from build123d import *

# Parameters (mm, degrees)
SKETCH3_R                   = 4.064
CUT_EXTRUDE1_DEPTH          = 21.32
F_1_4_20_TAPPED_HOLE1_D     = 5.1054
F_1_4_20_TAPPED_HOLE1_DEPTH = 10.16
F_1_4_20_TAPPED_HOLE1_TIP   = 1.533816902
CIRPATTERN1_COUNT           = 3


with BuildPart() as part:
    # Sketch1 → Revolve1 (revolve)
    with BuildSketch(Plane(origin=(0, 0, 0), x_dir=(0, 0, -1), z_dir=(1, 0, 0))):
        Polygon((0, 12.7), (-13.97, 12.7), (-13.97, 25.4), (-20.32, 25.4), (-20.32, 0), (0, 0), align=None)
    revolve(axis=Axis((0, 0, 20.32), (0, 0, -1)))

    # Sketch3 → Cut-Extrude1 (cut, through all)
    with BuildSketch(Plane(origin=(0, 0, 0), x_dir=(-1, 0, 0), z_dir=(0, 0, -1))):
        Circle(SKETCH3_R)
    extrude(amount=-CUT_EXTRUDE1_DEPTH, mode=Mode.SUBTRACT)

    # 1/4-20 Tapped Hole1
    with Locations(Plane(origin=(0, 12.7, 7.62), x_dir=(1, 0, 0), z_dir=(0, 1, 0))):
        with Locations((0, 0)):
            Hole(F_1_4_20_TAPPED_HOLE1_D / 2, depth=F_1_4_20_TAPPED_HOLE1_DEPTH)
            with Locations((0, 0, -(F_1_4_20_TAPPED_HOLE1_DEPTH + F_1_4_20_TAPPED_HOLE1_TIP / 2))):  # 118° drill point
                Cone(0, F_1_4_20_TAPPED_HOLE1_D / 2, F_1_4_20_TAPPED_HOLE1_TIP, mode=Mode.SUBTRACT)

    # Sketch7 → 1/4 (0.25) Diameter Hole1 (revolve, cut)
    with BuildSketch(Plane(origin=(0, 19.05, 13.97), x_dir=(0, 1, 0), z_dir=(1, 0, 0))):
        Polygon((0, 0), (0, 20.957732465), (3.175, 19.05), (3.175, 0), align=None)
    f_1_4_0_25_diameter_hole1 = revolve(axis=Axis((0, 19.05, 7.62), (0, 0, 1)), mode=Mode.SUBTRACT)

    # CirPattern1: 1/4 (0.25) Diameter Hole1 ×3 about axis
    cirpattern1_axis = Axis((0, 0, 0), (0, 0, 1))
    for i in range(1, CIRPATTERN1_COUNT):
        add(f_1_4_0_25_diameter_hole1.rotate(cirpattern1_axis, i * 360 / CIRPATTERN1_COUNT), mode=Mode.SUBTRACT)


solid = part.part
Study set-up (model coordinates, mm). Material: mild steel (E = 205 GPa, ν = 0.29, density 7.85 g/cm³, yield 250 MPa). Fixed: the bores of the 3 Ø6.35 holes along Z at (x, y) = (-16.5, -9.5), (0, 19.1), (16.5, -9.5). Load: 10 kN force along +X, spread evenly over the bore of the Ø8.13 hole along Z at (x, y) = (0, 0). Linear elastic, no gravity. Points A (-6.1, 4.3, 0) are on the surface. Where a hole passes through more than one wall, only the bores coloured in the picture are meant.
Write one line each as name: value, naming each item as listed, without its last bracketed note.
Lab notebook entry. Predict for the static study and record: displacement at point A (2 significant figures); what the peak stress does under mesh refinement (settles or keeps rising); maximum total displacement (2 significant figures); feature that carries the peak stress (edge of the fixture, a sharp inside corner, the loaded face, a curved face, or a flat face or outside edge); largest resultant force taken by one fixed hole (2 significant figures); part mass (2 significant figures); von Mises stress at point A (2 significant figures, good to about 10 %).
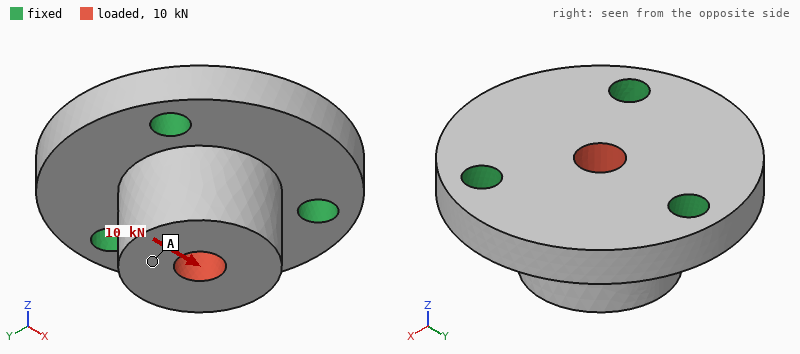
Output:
displacement at point A: 9.0 µm
what the peak stress does under mesh refinement: keeps rising
maximum total displacement: 9.6 µm
feature that carries the peak stress: edge of the fixture
largest resultant force taken by one fixed hole: 4.3 kN
part mass: 140 g
von Mises stress at point A: 17 MPa
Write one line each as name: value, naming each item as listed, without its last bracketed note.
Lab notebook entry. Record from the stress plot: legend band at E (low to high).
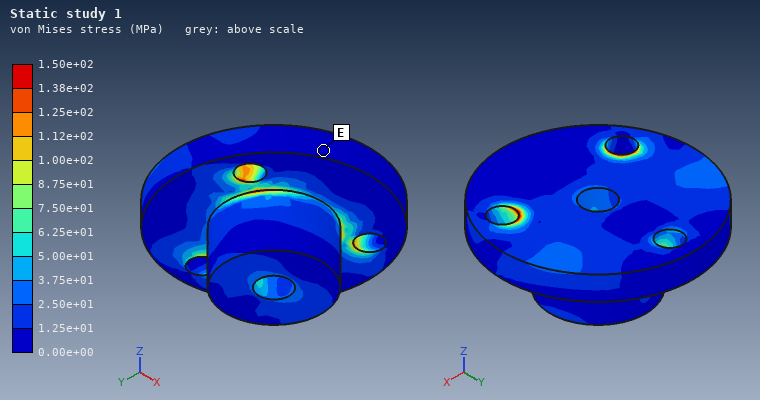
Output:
legend band at E: 0.00e+00 to 1.25e+01 MPa
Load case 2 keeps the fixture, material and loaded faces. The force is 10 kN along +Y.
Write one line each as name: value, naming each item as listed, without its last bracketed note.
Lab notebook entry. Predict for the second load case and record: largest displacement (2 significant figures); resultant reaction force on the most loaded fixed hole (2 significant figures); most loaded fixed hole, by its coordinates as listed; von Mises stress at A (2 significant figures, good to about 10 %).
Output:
largest displacement: 9.9 µm
resultant reaction force on the most loaded fixed hole: 4.7 kN
most loaded fixed hole, by its coordinates as listed: (0, 19.1)
von Mises stress at A: 16 MPa
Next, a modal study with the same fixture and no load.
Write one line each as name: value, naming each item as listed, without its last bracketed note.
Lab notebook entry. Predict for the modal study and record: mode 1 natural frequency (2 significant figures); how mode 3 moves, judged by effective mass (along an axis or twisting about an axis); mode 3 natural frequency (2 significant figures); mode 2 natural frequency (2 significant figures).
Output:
mode 1 natural frequency: 18 kHz
how mode 3 moves, judged by effective mass: along Z
mode 3 natural frequency: 21 kHz
mode 2 natural frequency: 18 kHz
